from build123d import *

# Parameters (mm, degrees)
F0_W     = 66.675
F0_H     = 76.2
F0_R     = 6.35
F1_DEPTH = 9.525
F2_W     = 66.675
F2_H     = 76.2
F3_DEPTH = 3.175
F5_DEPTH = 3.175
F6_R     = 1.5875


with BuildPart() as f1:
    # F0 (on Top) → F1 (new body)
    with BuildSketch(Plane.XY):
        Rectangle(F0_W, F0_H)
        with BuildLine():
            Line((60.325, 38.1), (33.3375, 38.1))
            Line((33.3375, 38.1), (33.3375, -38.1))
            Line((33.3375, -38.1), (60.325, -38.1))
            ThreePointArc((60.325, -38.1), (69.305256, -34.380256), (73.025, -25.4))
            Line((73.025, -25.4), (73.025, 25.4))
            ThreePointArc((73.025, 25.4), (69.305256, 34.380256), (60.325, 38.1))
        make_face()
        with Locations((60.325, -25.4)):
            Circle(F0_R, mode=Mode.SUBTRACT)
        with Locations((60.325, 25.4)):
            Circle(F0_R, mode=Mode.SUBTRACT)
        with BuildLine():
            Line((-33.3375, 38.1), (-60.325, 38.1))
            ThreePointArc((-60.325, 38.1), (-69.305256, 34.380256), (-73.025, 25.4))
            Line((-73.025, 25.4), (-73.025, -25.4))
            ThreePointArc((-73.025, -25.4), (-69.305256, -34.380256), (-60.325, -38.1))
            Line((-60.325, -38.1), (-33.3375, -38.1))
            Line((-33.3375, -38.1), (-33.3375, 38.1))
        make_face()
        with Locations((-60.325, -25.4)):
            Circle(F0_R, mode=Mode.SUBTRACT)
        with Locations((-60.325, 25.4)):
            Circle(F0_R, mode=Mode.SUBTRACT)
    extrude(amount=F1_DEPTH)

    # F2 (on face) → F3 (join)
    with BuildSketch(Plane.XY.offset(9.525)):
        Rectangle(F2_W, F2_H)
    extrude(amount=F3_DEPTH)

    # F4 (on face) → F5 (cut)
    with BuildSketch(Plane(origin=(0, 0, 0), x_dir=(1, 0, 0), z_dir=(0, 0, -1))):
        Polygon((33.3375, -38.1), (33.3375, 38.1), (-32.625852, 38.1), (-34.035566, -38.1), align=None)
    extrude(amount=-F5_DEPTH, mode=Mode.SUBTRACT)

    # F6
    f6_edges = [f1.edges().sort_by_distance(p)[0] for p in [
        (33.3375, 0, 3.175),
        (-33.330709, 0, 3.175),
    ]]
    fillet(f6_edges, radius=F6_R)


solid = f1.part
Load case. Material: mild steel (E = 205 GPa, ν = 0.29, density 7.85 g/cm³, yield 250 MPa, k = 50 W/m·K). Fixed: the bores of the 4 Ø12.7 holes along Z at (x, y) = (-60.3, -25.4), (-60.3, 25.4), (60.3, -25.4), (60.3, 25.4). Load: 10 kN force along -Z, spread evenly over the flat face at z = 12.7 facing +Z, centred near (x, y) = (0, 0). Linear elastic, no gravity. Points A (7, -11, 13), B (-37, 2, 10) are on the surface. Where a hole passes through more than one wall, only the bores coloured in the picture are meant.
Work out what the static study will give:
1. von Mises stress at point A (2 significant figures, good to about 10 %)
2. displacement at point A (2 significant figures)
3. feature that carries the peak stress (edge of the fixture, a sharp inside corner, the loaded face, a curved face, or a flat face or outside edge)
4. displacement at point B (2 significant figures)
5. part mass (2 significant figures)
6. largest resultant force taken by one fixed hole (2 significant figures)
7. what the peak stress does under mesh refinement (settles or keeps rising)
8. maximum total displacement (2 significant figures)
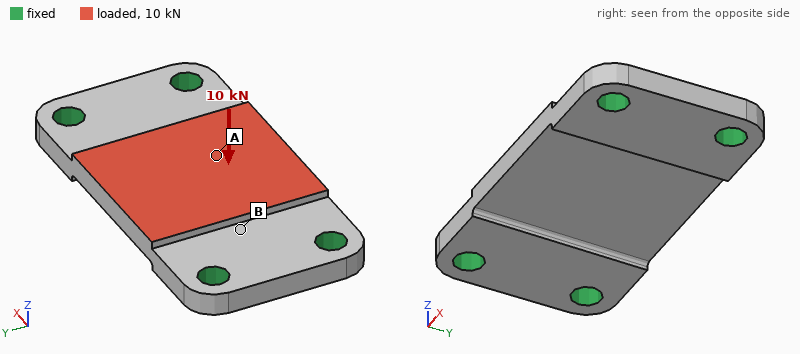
58 MPa
46 µm
edge of the fixture
18 µm
780 g
4.9 kN
keeps rising
50 µm
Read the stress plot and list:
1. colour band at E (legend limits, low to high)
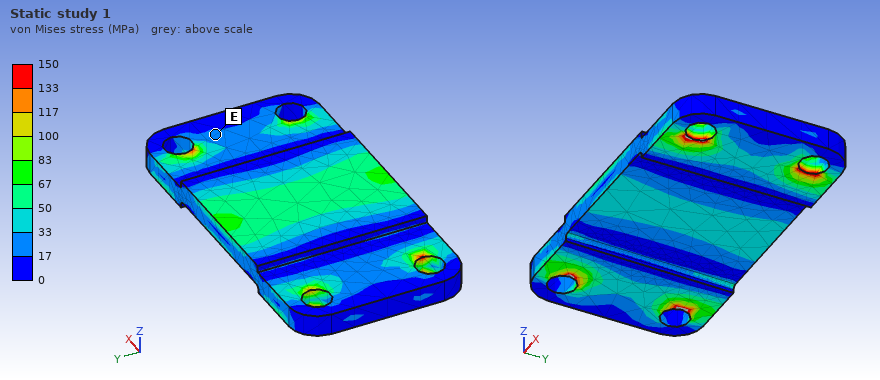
17 to 33 MPa
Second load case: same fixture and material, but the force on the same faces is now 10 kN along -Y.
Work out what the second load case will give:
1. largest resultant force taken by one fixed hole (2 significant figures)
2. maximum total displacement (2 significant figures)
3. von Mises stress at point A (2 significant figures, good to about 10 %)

3.7 kN
16 µm
8.4 MPa
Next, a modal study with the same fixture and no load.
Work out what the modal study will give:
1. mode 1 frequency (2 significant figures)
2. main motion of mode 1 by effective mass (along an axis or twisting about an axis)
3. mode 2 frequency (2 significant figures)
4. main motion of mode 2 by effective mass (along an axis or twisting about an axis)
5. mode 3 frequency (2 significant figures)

3900 Hz
along Z
5300 Hz
twisting about X
8900 Hz
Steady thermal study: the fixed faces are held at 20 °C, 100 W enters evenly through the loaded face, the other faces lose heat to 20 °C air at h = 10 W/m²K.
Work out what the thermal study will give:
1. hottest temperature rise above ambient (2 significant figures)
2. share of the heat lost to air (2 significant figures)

61 K
5.3 %
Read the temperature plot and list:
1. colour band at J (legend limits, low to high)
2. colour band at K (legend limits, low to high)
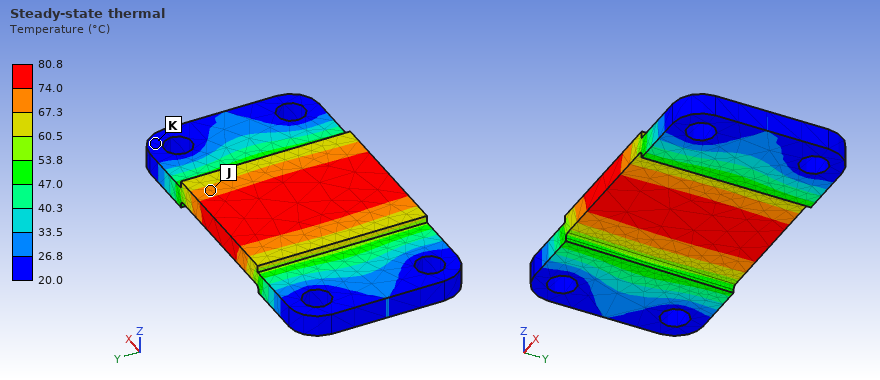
67.3 to 74.0 °C
20.0 to 26.8 °C
